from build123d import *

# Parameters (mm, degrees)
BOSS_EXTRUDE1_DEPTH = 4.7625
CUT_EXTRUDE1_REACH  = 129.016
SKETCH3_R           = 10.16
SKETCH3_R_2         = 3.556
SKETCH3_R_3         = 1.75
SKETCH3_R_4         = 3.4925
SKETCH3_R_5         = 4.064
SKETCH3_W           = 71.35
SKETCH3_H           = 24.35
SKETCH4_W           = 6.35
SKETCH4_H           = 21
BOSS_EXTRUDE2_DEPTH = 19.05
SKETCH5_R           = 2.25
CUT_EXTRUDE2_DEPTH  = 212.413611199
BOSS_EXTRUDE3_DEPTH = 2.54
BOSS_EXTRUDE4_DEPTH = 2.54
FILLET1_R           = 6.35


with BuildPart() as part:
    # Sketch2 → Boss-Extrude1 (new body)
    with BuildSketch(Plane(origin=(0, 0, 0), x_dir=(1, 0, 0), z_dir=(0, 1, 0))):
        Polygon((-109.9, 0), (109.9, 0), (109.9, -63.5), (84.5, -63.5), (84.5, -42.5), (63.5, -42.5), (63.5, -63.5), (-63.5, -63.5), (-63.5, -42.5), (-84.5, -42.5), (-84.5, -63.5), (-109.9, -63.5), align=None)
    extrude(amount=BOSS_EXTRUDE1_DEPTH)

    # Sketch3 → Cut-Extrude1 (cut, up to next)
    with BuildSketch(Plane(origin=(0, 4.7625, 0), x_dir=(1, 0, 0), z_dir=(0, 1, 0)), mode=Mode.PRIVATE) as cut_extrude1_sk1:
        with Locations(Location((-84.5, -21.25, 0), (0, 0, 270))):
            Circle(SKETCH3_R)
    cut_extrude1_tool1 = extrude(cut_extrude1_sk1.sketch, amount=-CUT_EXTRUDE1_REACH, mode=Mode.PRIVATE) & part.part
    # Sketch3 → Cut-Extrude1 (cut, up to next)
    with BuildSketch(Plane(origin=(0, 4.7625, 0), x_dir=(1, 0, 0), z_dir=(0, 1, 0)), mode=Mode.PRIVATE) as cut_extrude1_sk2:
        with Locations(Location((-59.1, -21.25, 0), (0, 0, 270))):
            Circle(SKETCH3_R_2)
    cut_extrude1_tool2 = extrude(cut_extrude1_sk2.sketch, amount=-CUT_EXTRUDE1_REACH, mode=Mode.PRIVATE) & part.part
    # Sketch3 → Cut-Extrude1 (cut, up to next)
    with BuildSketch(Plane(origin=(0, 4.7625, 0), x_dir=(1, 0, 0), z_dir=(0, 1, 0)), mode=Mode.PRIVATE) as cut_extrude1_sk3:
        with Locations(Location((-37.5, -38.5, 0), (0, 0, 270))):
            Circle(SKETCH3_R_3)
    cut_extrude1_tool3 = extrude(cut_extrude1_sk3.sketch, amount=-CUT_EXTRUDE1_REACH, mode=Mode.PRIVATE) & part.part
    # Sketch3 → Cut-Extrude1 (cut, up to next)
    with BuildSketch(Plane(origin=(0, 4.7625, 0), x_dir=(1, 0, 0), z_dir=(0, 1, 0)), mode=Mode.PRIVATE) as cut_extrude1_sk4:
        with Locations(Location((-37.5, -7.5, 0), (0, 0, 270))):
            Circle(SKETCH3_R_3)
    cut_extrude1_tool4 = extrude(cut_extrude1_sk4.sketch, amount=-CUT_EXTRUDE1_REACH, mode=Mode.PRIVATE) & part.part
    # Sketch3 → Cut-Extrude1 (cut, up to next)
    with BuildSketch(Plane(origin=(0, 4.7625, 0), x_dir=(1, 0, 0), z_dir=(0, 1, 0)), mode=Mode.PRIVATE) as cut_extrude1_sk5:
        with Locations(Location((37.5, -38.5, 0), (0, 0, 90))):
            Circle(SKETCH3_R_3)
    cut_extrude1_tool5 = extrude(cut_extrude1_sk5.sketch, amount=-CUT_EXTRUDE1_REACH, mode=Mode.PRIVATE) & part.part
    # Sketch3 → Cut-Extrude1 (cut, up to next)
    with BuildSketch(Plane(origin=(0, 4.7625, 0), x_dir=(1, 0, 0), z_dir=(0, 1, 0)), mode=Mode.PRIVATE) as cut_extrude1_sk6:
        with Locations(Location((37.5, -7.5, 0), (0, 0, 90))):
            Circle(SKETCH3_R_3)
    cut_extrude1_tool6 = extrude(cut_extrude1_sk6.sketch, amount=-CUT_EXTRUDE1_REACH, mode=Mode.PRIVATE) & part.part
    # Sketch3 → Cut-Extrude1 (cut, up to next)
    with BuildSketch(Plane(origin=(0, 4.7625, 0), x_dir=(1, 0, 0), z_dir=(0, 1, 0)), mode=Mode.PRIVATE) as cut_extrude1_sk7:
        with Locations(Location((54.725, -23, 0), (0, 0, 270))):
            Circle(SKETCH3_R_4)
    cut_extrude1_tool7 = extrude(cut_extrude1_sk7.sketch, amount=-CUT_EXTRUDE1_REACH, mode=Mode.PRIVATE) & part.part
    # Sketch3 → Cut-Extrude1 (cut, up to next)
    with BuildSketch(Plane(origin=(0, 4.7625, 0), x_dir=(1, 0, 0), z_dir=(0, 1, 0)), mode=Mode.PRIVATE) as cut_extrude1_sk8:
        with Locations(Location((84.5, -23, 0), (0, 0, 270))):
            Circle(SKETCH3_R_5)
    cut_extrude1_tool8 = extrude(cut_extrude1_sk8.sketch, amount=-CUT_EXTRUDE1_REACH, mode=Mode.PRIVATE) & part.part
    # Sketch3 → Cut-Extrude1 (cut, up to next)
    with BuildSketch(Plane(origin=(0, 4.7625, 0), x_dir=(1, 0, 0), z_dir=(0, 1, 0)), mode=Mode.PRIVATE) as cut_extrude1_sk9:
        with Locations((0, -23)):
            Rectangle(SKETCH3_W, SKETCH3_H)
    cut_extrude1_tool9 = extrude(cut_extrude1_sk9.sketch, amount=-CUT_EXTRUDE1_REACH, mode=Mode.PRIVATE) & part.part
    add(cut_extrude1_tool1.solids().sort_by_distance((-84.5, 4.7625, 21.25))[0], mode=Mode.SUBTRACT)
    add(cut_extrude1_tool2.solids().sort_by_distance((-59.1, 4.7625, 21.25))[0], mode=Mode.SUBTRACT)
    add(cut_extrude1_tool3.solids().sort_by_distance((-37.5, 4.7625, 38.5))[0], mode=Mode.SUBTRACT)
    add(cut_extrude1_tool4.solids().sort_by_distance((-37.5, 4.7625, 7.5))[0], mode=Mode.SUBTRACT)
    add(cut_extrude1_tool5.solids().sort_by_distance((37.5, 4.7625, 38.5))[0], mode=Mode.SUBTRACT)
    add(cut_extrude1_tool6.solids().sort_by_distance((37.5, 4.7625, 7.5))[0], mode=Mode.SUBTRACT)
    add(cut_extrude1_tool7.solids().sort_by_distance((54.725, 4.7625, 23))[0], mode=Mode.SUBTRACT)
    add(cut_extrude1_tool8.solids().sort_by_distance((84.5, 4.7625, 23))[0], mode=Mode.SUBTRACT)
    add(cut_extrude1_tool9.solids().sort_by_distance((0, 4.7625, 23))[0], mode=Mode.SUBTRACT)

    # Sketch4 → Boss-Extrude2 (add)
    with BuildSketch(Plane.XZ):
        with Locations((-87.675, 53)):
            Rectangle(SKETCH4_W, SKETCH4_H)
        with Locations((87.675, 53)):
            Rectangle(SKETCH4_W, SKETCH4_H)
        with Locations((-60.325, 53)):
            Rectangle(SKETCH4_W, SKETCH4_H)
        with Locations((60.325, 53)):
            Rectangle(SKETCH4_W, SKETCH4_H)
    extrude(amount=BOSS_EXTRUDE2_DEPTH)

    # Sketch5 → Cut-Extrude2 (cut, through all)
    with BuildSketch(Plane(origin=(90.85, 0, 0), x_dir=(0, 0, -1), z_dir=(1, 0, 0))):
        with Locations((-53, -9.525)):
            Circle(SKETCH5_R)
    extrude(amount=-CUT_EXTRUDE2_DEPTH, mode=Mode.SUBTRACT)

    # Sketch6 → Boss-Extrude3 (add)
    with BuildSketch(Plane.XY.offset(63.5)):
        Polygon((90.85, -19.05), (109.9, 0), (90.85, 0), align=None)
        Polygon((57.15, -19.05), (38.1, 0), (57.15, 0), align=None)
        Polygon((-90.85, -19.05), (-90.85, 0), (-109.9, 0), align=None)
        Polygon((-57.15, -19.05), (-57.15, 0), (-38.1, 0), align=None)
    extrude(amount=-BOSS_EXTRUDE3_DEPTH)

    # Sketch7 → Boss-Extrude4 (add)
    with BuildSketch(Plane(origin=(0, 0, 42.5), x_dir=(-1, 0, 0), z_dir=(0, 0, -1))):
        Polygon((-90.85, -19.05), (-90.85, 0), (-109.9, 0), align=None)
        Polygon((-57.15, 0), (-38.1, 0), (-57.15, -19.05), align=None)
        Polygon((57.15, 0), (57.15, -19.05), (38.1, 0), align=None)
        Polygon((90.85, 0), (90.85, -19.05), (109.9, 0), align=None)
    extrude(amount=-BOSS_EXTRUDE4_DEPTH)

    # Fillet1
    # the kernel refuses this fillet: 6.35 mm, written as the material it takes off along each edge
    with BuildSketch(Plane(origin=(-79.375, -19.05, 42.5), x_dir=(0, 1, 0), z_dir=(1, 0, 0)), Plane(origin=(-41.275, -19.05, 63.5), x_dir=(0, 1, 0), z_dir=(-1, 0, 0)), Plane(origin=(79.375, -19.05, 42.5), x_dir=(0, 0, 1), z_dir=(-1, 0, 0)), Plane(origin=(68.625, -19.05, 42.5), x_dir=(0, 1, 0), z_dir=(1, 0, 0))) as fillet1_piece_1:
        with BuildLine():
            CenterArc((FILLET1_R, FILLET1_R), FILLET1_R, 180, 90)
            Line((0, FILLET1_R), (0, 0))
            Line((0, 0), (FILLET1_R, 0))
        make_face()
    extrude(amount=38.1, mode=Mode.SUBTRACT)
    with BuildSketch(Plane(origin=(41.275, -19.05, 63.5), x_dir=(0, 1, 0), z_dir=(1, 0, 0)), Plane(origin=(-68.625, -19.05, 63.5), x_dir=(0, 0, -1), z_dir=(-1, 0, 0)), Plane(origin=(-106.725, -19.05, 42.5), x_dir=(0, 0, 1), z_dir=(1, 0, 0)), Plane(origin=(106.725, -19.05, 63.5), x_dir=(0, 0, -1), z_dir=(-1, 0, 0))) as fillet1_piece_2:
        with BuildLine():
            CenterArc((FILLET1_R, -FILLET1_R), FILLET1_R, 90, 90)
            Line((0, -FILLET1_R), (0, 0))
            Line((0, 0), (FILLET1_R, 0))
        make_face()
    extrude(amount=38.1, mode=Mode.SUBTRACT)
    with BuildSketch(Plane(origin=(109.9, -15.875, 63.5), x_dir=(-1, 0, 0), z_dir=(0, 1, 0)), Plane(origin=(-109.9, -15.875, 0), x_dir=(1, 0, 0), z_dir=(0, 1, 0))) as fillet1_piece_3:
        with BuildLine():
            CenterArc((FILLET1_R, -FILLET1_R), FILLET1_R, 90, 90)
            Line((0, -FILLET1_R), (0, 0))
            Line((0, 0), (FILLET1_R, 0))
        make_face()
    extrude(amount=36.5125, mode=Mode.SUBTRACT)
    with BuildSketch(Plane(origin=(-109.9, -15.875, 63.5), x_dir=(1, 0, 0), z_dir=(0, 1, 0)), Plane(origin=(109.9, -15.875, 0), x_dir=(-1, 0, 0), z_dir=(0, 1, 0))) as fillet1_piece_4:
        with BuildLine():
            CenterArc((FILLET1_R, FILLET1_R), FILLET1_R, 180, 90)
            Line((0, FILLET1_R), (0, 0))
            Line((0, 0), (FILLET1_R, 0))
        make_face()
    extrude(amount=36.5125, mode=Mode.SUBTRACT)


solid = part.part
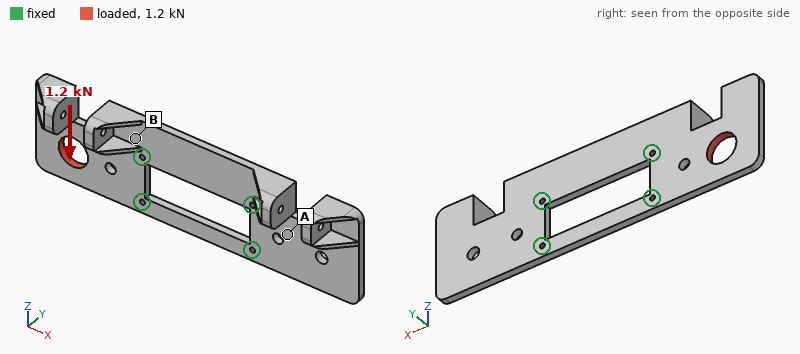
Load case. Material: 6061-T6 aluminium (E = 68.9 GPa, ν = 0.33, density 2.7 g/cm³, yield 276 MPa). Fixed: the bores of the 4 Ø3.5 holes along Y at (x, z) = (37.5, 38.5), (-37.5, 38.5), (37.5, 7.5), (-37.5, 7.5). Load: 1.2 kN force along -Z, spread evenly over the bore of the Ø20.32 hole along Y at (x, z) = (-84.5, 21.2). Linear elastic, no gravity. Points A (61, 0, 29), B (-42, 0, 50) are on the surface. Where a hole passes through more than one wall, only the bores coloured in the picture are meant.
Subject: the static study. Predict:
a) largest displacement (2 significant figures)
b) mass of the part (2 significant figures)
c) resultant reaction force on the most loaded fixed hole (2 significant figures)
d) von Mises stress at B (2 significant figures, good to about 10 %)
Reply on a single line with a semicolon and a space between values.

57 µm; 170 g; 1.4 kN; 9.1 MPa
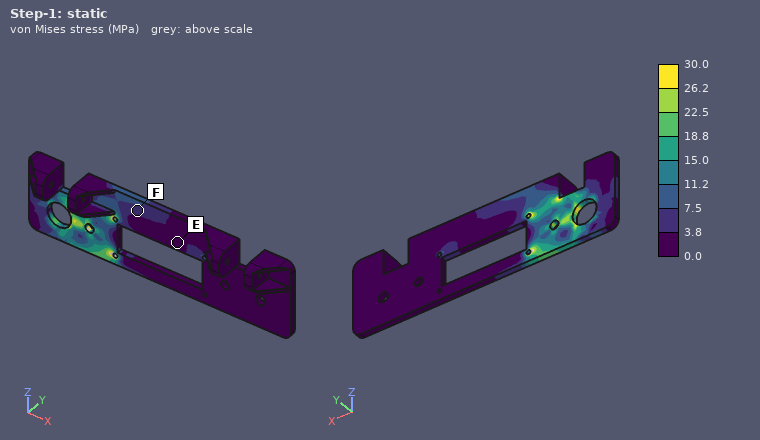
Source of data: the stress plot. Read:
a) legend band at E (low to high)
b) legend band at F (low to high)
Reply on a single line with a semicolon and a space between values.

0.0 to 3.8 MPa; 3.8 to 7.5 MPa
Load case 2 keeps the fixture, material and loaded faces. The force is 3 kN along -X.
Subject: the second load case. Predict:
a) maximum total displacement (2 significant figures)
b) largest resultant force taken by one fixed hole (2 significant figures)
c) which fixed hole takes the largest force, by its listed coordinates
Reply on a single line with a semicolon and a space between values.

20 µm; 1.7 kN; (-37.5, 7.5)
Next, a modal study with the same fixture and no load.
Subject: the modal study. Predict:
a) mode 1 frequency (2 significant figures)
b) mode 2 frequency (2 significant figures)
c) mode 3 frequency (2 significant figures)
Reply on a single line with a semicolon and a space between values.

580 Hz; 590 Hz; 1200 Hz
